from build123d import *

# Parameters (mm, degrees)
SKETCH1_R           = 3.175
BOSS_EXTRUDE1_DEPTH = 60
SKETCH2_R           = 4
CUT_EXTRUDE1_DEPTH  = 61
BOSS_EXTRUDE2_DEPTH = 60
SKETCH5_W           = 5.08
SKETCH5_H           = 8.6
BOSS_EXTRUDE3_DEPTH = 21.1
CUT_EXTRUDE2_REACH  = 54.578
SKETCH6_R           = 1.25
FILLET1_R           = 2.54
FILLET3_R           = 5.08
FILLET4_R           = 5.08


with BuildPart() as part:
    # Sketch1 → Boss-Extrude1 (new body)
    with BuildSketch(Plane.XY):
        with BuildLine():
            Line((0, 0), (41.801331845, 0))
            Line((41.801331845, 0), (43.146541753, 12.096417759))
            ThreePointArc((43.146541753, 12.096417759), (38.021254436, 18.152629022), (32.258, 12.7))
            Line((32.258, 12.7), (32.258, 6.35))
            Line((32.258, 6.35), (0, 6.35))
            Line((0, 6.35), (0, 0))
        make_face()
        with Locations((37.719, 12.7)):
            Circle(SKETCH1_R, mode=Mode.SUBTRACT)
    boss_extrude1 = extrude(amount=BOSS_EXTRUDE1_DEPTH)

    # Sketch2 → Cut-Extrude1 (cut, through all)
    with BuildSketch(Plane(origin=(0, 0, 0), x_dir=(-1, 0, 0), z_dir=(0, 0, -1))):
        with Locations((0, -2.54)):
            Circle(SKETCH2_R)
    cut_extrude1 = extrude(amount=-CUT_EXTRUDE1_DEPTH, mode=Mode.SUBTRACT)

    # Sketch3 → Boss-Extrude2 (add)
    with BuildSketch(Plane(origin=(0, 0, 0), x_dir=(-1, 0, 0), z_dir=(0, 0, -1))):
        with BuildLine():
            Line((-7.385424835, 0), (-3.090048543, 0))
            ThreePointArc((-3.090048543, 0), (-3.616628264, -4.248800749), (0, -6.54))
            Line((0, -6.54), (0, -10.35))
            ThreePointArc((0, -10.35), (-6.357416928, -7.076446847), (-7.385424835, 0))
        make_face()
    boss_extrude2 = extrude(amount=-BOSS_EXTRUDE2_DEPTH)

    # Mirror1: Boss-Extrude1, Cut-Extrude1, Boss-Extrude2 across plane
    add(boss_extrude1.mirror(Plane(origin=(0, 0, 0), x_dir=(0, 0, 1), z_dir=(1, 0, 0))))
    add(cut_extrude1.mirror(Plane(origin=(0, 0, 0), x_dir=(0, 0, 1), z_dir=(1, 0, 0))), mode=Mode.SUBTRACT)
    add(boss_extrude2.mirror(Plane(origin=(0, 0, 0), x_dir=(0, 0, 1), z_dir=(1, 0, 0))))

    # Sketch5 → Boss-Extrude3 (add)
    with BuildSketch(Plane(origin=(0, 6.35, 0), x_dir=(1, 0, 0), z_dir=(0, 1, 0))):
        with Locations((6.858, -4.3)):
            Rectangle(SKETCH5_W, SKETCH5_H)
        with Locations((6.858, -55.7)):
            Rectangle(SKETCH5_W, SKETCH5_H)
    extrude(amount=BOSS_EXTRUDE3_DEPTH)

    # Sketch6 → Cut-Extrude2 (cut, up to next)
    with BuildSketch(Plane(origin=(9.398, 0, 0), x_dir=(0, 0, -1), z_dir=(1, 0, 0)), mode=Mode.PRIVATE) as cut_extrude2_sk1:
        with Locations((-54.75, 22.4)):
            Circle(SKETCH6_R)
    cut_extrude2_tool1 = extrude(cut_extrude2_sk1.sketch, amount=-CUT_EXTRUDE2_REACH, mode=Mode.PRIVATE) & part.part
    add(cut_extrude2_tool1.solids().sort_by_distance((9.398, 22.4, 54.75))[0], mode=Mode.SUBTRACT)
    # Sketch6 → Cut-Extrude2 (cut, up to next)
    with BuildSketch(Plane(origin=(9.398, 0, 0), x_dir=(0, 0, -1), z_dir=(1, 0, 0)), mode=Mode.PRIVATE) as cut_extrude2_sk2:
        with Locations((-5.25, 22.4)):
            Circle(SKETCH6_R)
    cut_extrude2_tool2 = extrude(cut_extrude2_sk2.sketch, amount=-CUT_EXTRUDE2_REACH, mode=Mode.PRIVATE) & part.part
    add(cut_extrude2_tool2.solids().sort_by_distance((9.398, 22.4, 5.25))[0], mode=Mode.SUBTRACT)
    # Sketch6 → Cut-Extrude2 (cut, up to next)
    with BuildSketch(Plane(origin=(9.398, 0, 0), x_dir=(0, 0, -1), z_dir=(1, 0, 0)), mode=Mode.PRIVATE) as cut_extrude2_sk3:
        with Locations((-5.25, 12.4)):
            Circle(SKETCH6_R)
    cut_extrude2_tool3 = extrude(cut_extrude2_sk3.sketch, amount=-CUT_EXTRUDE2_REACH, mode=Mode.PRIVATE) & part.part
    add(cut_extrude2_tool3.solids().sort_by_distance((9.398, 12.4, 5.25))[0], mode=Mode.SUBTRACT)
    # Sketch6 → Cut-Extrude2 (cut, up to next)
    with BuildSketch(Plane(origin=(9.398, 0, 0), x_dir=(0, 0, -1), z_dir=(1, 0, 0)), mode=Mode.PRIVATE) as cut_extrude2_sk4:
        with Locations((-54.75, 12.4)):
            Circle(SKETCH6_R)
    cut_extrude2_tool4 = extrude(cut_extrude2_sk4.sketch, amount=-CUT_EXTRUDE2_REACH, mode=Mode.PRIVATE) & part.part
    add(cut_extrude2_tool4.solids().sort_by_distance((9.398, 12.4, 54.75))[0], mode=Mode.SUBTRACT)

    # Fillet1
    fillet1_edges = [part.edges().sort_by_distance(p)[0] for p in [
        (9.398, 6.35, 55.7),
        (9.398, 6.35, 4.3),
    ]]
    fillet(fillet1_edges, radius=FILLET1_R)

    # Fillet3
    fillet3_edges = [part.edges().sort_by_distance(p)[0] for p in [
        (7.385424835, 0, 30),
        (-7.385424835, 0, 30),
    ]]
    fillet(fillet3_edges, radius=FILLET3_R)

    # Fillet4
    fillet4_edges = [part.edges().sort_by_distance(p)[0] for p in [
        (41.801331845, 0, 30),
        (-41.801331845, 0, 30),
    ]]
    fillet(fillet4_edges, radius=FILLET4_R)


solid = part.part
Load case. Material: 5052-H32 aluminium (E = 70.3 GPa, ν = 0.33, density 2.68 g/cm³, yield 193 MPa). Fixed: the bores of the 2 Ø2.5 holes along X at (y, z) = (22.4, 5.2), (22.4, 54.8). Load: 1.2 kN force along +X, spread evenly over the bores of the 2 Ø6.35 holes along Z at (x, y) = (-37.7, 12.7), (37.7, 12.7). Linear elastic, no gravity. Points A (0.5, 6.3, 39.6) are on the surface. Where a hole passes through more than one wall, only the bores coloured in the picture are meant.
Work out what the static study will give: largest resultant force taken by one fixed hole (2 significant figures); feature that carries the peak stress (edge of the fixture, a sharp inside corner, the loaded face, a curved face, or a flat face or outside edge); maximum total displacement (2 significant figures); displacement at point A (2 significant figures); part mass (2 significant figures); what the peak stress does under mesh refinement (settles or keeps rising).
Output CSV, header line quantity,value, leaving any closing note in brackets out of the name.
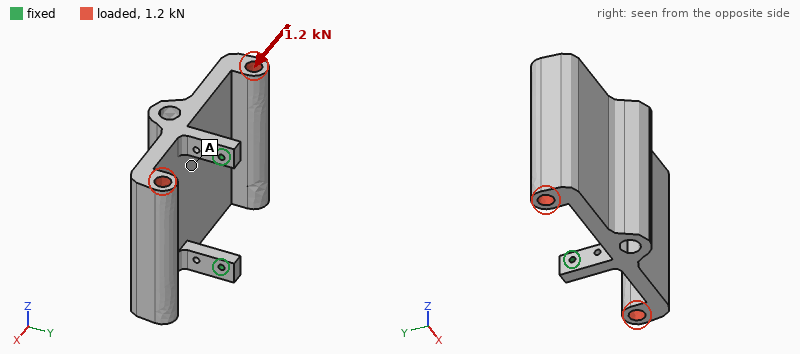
quantity,value
largest resultant force taken by one fixed hole,600 N
feature that carries the peak stress,edge of the fixture
maximum total displacement,92 µm
displacement at point A,64 µm
part mass,130 g
what the peak stress does under mesh refinement,keeps rising
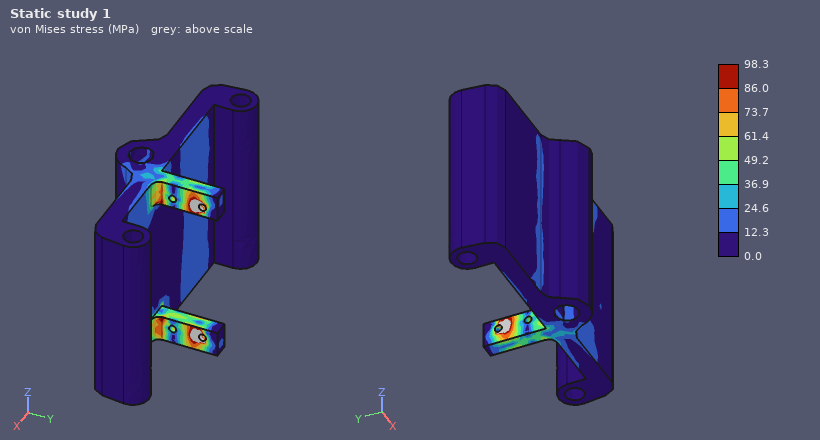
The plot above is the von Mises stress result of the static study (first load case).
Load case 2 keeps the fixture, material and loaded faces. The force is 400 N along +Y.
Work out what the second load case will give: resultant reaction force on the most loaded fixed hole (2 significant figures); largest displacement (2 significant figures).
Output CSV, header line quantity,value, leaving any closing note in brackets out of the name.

quantity,value
resultant reaction force on the most loaded fixed hole,200 N
largest displacement,0.24 mm
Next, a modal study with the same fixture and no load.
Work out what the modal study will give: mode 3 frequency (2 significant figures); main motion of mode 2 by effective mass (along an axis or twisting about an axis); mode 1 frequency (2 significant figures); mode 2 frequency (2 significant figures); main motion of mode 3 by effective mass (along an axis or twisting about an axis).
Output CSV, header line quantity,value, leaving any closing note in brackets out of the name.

quantity,value
mode 3 frequency,2100 Hz
main motion of mode 2 by effective mass,along Z
mode 1 frequency,400 Hz
mode 2 frequency,1600 Hz
main motion of mode 3 by effective mass,along X
